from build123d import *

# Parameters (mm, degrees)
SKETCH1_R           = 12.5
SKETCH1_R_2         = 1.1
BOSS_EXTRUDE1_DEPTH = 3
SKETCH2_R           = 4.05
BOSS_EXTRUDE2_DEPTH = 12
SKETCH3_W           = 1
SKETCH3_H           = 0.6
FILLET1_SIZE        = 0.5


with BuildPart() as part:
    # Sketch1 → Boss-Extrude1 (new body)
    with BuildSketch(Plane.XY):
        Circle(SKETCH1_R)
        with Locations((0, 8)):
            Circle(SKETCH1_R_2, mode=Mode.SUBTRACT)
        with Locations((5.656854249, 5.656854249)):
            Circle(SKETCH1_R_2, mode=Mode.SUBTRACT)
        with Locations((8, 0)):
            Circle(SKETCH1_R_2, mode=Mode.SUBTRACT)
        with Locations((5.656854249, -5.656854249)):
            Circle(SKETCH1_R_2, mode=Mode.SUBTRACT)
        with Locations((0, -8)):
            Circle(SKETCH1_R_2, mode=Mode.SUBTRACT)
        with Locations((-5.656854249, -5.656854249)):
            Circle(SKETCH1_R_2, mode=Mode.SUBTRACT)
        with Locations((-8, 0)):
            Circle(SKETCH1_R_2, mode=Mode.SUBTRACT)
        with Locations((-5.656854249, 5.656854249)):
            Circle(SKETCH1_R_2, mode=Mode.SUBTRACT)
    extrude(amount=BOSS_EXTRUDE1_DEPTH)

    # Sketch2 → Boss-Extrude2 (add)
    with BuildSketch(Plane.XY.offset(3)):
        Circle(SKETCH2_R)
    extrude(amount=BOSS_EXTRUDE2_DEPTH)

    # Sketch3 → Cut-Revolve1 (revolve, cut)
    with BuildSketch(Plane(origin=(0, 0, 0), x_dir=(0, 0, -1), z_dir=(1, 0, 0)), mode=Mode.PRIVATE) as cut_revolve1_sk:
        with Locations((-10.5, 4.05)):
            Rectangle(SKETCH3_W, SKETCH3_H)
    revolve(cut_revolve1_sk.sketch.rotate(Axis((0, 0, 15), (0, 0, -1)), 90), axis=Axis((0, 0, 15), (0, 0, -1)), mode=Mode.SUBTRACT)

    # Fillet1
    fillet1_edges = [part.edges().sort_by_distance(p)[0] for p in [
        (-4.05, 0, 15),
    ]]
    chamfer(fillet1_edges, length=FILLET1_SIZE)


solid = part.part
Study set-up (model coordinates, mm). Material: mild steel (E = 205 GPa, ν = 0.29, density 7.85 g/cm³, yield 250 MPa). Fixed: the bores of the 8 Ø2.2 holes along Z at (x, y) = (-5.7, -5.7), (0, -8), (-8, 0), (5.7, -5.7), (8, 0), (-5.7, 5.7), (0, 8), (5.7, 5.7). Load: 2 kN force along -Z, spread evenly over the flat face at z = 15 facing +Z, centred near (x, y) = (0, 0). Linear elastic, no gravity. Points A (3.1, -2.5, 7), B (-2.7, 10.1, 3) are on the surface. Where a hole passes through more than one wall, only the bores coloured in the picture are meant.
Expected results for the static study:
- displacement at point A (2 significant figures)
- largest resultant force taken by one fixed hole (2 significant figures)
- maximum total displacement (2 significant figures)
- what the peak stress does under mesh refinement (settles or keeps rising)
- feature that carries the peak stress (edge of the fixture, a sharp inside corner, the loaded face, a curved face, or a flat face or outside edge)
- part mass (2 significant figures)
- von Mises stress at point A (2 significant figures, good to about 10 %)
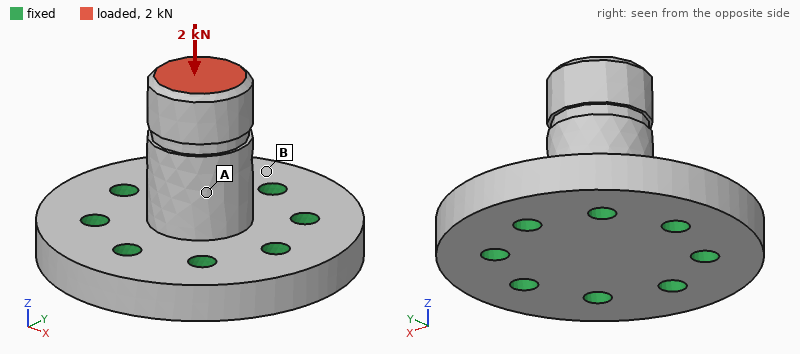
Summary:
2.9 µm
270 N
4.7 µm
keeps rising
edge of the fixture
16 g
36 MPa
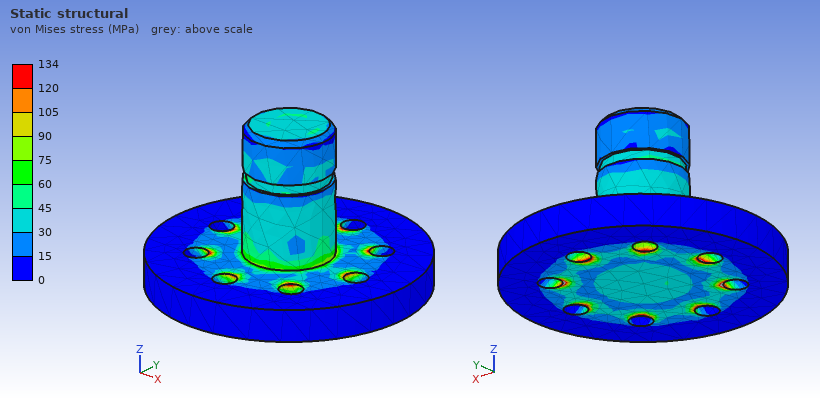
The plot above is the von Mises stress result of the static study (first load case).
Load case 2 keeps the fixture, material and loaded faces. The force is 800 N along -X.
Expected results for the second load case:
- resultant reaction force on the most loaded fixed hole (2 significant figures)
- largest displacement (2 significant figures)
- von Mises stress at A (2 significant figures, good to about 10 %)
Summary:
480 N
24 µm
95 MPa
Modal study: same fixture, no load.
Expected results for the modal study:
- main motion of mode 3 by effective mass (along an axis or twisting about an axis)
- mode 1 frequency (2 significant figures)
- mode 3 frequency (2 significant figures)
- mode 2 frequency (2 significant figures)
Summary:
along Z
24 kHz
54 kHz
24 kHz
